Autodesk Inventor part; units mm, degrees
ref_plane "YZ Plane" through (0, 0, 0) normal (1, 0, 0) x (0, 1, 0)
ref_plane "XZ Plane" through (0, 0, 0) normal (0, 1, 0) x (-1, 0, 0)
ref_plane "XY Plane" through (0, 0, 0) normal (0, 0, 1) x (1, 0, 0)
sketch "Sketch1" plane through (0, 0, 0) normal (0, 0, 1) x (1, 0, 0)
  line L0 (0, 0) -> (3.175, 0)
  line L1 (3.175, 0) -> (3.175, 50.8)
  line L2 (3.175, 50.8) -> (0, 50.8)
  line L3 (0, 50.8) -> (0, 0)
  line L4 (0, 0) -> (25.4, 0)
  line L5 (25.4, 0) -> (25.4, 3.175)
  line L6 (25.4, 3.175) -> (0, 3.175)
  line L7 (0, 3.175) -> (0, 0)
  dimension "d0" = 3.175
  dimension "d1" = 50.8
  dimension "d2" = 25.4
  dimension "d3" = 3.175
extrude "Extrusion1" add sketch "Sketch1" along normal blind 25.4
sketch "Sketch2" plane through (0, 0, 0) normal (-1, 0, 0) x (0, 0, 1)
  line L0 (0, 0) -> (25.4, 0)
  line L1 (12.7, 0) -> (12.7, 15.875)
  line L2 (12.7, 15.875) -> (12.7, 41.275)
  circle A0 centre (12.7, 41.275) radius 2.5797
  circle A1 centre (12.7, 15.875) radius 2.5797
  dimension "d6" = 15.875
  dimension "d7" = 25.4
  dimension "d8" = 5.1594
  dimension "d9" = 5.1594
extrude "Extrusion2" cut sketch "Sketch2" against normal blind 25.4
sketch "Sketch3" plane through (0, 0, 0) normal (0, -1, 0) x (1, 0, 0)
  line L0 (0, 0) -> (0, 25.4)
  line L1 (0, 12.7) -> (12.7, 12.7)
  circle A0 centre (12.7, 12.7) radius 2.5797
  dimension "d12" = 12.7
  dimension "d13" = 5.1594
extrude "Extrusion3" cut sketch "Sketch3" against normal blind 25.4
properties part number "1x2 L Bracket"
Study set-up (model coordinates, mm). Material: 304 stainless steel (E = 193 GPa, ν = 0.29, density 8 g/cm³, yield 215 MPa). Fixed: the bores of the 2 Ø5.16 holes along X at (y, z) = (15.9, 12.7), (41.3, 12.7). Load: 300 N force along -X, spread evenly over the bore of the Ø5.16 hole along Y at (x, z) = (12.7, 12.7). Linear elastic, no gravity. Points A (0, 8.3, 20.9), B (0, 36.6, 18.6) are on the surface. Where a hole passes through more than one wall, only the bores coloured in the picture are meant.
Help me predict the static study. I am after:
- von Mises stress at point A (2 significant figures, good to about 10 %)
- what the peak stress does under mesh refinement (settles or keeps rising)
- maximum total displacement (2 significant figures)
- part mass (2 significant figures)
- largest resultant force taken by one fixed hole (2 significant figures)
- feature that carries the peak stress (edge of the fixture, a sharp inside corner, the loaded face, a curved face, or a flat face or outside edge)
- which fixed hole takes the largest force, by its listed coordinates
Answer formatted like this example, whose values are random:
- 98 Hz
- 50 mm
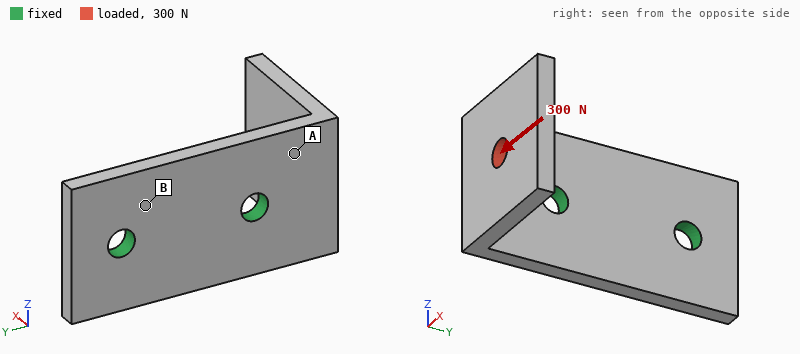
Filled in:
- 41 MPa
- keeps rising
- 57 µm
- 46 g
- 330 N
- edge of the fixture
- (15.9, 12.7)
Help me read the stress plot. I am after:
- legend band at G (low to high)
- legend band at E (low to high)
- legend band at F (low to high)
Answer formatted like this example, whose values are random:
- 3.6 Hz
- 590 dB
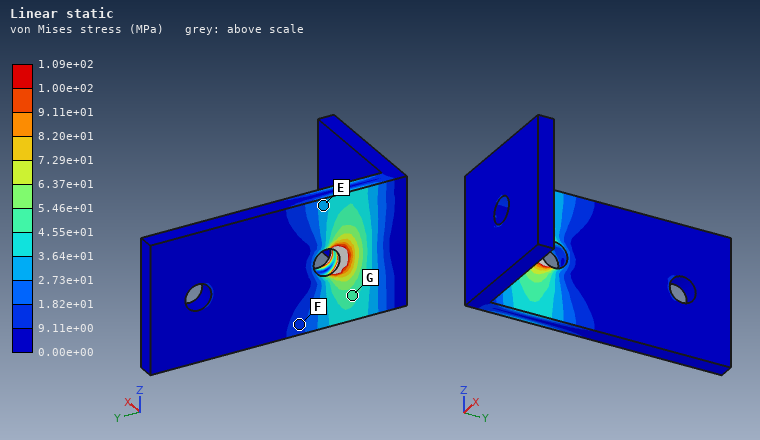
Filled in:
- 4.55e+01 to 5.46e+01 MPa
- 2.73e+01 to 3.64e+01 MPa
- 9.11e+00 to 1.82e+01 MPa
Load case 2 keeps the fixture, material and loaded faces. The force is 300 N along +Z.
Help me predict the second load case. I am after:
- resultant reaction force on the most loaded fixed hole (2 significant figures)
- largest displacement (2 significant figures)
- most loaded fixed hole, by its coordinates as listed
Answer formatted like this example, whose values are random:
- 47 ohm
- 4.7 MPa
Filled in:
- 410 N
- 51 µm
- (15.9, 12.7)
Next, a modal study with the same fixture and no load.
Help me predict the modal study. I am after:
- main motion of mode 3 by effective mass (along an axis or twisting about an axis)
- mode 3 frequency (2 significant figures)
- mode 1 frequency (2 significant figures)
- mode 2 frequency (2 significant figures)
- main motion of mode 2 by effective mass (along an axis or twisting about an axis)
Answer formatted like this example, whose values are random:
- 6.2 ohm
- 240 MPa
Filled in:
- along X
- 7000 Hz
- 2300 Hz
- 3400 Hz
- along Z
